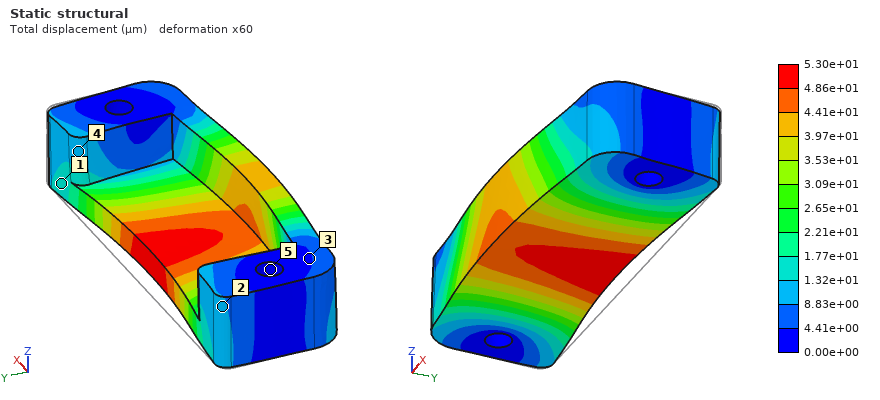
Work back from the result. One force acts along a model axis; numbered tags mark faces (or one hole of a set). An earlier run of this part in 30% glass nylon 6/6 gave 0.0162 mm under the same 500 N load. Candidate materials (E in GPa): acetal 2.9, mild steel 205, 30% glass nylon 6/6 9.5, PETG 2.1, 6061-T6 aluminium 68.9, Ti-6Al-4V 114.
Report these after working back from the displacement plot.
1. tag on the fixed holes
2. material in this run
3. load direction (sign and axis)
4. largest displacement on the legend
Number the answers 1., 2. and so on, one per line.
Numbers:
1. 5
2. acetal
3. -Y
4. 5.30e+01 µm
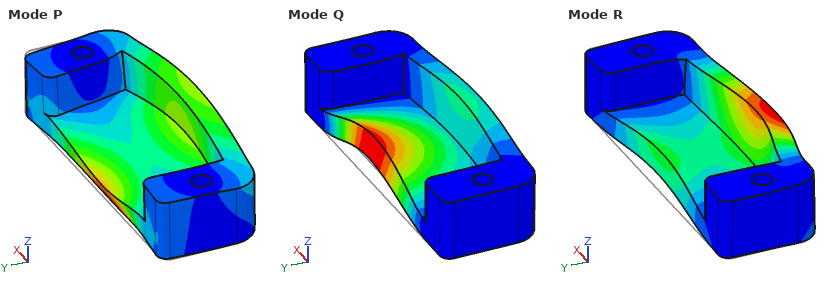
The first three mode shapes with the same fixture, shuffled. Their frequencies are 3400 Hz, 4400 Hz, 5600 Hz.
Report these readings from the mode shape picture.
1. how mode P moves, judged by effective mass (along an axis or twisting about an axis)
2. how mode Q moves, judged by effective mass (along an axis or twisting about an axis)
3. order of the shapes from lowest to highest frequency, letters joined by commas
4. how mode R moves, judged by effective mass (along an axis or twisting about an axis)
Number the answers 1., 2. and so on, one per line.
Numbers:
1. along Y
2. along Z
3. Q, R, P
4. along Y
